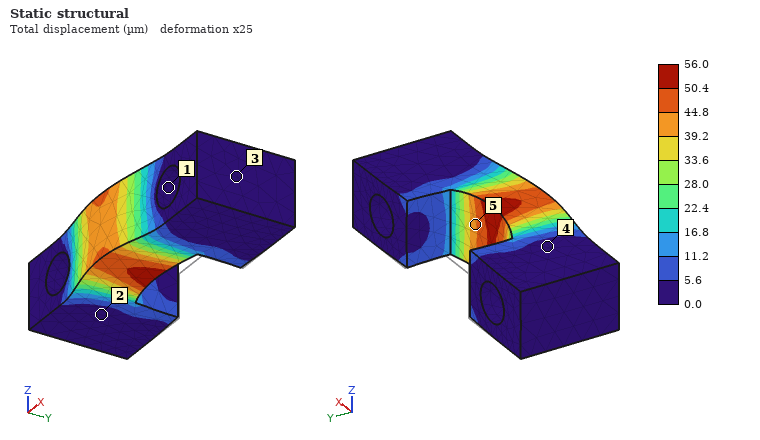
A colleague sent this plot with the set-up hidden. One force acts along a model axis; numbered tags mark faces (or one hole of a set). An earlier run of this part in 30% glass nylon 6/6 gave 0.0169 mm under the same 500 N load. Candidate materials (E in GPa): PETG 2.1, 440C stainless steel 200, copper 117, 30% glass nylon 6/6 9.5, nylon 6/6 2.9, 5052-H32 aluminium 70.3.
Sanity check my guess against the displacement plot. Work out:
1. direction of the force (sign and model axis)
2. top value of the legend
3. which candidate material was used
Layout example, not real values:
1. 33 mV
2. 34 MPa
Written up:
1. -Y
2. 56.0 µm
3. nylon 6/6
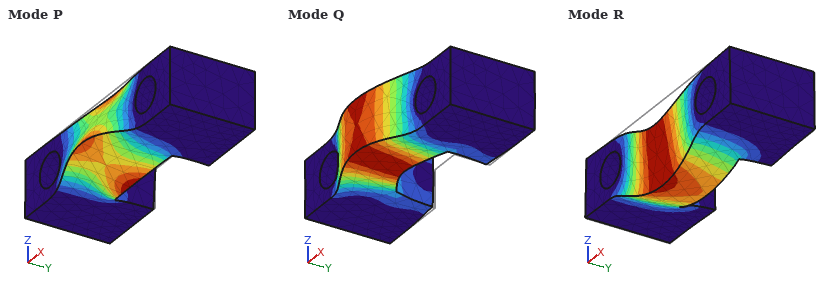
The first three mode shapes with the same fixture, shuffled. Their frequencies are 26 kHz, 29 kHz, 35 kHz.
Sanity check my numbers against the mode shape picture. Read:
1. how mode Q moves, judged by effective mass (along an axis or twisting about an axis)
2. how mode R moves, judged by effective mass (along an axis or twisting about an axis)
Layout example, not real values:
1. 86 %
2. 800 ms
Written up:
1. along Y
2. along Z
